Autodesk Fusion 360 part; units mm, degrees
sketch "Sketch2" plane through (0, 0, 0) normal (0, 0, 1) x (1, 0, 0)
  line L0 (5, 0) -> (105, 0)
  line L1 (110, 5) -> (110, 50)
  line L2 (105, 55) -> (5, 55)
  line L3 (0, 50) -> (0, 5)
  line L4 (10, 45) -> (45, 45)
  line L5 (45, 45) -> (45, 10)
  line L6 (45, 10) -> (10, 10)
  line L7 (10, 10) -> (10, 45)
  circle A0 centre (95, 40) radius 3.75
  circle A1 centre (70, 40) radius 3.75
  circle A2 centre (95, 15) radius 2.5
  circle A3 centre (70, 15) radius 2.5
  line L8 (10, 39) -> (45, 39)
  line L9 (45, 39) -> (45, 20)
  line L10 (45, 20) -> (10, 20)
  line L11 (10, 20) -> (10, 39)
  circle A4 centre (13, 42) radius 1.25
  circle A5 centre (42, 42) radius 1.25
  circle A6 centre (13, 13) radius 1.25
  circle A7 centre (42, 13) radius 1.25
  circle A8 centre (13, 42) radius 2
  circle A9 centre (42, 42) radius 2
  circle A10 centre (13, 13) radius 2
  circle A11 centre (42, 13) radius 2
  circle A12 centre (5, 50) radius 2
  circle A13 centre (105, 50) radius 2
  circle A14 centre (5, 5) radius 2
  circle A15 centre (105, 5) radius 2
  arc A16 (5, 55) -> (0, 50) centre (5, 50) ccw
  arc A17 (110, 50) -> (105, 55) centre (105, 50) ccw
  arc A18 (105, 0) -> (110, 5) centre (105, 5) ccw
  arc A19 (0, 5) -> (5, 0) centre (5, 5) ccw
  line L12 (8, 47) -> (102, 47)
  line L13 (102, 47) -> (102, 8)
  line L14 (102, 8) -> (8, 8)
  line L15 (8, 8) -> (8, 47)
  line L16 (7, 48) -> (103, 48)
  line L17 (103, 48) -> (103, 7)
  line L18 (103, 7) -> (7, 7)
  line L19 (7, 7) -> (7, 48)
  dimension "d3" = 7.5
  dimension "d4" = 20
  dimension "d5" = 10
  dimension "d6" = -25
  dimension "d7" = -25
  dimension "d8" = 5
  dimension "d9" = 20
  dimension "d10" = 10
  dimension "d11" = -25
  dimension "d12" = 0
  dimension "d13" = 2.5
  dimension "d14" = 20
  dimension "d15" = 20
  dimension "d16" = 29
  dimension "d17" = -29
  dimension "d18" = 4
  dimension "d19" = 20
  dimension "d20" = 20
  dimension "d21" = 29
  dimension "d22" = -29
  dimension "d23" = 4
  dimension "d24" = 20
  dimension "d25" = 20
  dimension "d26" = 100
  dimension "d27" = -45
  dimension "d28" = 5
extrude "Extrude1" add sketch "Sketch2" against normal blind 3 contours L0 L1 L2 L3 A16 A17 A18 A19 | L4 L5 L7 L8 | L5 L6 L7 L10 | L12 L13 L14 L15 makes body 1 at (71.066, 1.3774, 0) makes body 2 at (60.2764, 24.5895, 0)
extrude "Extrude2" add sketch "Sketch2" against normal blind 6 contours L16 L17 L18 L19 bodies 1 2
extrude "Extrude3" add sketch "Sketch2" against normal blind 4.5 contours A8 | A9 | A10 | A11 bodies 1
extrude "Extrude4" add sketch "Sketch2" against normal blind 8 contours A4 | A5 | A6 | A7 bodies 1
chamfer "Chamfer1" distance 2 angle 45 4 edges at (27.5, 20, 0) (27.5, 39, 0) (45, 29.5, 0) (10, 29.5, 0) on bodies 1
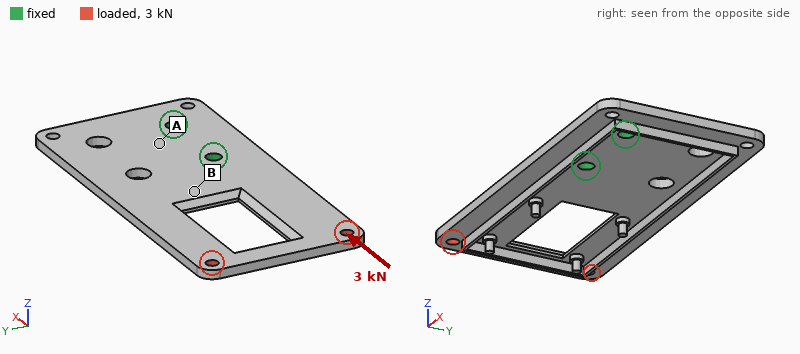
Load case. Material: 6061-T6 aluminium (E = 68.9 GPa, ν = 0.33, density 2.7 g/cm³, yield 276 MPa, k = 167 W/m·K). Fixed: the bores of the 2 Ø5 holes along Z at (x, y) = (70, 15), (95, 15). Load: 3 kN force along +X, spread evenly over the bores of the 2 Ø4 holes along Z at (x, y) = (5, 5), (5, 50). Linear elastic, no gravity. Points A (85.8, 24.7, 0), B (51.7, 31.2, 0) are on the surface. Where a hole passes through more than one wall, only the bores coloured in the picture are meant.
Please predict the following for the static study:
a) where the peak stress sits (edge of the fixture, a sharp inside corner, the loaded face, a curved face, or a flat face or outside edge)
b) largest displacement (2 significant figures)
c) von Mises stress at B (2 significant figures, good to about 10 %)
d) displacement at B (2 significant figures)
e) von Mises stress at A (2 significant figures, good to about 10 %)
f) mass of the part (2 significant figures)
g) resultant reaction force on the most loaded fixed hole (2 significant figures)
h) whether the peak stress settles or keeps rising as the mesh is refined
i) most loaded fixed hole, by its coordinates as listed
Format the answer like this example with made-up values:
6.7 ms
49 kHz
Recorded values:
edge of the fixture
0.14 mm
11 MPa
0.024 mm
27 MPa
44 g
2.4 kN
keeps rising
(70, 15)
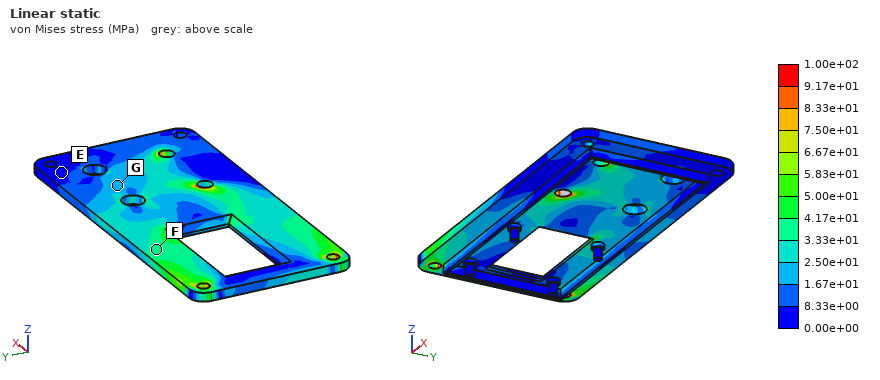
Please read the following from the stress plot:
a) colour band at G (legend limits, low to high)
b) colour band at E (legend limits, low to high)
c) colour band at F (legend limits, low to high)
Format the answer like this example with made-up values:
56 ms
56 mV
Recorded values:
1.67e+01 to 2.50e+01 MPa
0.00e+00 to 8.33e+00 MPa
3.33e+01 to 4.17e+01 MPa
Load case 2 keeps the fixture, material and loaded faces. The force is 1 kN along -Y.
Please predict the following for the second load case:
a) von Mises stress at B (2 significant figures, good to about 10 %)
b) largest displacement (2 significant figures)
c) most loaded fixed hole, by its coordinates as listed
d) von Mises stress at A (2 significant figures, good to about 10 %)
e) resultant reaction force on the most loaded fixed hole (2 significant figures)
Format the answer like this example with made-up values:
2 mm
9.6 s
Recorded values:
27 MPa
0.25 mm
(70, 15)
34 MPa
3.2 kN
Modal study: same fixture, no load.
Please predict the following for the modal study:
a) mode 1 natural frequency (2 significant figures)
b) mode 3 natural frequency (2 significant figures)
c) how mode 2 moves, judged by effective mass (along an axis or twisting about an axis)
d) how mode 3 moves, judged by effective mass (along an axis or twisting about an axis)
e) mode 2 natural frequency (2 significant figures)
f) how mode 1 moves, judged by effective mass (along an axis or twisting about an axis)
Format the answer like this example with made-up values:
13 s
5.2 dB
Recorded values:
540 Hz
1900 Hz
twisting about X
along Z
1000 Hz
along Z
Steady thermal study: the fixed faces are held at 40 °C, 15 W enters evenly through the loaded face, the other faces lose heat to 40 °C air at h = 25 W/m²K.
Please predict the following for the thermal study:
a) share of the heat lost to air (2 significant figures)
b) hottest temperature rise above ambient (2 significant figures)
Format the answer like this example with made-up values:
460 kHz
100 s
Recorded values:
32 %
48 K
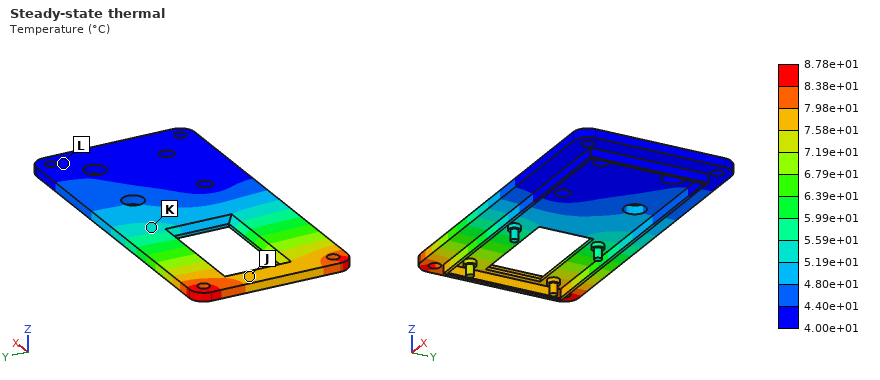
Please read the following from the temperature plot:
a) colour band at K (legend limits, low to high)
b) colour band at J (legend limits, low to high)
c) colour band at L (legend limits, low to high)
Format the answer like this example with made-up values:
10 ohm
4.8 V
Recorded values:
5.19e+01 to 5.59e+01 °C
7.58e+01 to 7.98e+01 °C
4.00e+01 to 4.40e+01 °C
